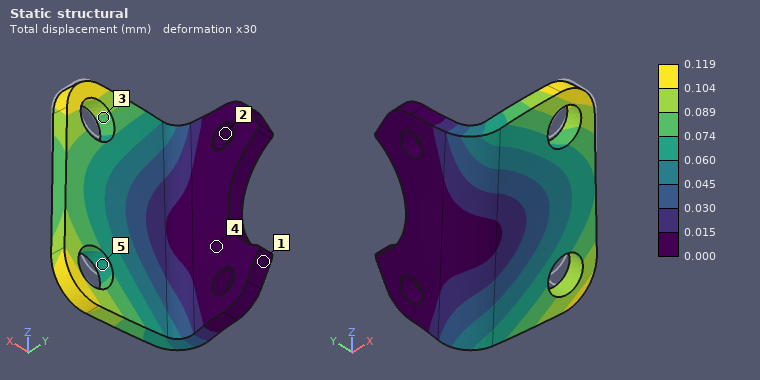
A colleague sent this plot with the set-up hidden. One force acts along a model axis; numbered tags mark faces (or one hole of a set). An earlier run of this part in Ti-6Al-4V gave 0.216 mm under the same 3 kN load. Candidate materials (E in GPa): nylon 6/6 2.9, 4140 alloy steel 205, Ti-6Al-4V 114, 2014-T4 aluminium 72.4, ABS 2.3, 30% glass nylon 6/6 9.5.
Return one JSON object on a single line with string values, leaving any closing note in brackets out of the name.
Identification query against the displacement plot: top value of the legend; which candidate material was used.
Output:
{"top value of the legend": "0.119 mm", "which candidate material was used": "4140 alloy steel"}
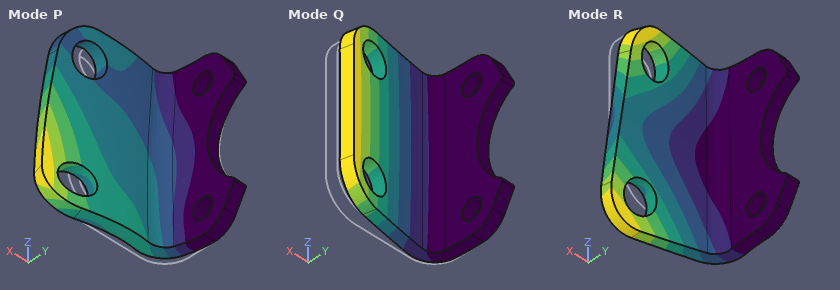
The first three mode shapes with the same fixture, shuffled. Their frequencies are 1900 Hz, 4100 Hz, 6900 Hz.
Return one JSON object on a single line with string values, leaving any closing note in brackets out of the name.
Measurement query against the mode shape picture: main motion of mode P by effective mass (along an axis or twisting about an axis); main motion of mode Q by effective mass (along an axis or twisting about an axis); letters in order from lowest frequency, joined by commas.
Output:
{"main motion of mode P by effective mass": "along X", "main motion of mode Q by effective mass": "along Y", "letters in order from lowest frequency, joined by commas": "Q, R, P"}
